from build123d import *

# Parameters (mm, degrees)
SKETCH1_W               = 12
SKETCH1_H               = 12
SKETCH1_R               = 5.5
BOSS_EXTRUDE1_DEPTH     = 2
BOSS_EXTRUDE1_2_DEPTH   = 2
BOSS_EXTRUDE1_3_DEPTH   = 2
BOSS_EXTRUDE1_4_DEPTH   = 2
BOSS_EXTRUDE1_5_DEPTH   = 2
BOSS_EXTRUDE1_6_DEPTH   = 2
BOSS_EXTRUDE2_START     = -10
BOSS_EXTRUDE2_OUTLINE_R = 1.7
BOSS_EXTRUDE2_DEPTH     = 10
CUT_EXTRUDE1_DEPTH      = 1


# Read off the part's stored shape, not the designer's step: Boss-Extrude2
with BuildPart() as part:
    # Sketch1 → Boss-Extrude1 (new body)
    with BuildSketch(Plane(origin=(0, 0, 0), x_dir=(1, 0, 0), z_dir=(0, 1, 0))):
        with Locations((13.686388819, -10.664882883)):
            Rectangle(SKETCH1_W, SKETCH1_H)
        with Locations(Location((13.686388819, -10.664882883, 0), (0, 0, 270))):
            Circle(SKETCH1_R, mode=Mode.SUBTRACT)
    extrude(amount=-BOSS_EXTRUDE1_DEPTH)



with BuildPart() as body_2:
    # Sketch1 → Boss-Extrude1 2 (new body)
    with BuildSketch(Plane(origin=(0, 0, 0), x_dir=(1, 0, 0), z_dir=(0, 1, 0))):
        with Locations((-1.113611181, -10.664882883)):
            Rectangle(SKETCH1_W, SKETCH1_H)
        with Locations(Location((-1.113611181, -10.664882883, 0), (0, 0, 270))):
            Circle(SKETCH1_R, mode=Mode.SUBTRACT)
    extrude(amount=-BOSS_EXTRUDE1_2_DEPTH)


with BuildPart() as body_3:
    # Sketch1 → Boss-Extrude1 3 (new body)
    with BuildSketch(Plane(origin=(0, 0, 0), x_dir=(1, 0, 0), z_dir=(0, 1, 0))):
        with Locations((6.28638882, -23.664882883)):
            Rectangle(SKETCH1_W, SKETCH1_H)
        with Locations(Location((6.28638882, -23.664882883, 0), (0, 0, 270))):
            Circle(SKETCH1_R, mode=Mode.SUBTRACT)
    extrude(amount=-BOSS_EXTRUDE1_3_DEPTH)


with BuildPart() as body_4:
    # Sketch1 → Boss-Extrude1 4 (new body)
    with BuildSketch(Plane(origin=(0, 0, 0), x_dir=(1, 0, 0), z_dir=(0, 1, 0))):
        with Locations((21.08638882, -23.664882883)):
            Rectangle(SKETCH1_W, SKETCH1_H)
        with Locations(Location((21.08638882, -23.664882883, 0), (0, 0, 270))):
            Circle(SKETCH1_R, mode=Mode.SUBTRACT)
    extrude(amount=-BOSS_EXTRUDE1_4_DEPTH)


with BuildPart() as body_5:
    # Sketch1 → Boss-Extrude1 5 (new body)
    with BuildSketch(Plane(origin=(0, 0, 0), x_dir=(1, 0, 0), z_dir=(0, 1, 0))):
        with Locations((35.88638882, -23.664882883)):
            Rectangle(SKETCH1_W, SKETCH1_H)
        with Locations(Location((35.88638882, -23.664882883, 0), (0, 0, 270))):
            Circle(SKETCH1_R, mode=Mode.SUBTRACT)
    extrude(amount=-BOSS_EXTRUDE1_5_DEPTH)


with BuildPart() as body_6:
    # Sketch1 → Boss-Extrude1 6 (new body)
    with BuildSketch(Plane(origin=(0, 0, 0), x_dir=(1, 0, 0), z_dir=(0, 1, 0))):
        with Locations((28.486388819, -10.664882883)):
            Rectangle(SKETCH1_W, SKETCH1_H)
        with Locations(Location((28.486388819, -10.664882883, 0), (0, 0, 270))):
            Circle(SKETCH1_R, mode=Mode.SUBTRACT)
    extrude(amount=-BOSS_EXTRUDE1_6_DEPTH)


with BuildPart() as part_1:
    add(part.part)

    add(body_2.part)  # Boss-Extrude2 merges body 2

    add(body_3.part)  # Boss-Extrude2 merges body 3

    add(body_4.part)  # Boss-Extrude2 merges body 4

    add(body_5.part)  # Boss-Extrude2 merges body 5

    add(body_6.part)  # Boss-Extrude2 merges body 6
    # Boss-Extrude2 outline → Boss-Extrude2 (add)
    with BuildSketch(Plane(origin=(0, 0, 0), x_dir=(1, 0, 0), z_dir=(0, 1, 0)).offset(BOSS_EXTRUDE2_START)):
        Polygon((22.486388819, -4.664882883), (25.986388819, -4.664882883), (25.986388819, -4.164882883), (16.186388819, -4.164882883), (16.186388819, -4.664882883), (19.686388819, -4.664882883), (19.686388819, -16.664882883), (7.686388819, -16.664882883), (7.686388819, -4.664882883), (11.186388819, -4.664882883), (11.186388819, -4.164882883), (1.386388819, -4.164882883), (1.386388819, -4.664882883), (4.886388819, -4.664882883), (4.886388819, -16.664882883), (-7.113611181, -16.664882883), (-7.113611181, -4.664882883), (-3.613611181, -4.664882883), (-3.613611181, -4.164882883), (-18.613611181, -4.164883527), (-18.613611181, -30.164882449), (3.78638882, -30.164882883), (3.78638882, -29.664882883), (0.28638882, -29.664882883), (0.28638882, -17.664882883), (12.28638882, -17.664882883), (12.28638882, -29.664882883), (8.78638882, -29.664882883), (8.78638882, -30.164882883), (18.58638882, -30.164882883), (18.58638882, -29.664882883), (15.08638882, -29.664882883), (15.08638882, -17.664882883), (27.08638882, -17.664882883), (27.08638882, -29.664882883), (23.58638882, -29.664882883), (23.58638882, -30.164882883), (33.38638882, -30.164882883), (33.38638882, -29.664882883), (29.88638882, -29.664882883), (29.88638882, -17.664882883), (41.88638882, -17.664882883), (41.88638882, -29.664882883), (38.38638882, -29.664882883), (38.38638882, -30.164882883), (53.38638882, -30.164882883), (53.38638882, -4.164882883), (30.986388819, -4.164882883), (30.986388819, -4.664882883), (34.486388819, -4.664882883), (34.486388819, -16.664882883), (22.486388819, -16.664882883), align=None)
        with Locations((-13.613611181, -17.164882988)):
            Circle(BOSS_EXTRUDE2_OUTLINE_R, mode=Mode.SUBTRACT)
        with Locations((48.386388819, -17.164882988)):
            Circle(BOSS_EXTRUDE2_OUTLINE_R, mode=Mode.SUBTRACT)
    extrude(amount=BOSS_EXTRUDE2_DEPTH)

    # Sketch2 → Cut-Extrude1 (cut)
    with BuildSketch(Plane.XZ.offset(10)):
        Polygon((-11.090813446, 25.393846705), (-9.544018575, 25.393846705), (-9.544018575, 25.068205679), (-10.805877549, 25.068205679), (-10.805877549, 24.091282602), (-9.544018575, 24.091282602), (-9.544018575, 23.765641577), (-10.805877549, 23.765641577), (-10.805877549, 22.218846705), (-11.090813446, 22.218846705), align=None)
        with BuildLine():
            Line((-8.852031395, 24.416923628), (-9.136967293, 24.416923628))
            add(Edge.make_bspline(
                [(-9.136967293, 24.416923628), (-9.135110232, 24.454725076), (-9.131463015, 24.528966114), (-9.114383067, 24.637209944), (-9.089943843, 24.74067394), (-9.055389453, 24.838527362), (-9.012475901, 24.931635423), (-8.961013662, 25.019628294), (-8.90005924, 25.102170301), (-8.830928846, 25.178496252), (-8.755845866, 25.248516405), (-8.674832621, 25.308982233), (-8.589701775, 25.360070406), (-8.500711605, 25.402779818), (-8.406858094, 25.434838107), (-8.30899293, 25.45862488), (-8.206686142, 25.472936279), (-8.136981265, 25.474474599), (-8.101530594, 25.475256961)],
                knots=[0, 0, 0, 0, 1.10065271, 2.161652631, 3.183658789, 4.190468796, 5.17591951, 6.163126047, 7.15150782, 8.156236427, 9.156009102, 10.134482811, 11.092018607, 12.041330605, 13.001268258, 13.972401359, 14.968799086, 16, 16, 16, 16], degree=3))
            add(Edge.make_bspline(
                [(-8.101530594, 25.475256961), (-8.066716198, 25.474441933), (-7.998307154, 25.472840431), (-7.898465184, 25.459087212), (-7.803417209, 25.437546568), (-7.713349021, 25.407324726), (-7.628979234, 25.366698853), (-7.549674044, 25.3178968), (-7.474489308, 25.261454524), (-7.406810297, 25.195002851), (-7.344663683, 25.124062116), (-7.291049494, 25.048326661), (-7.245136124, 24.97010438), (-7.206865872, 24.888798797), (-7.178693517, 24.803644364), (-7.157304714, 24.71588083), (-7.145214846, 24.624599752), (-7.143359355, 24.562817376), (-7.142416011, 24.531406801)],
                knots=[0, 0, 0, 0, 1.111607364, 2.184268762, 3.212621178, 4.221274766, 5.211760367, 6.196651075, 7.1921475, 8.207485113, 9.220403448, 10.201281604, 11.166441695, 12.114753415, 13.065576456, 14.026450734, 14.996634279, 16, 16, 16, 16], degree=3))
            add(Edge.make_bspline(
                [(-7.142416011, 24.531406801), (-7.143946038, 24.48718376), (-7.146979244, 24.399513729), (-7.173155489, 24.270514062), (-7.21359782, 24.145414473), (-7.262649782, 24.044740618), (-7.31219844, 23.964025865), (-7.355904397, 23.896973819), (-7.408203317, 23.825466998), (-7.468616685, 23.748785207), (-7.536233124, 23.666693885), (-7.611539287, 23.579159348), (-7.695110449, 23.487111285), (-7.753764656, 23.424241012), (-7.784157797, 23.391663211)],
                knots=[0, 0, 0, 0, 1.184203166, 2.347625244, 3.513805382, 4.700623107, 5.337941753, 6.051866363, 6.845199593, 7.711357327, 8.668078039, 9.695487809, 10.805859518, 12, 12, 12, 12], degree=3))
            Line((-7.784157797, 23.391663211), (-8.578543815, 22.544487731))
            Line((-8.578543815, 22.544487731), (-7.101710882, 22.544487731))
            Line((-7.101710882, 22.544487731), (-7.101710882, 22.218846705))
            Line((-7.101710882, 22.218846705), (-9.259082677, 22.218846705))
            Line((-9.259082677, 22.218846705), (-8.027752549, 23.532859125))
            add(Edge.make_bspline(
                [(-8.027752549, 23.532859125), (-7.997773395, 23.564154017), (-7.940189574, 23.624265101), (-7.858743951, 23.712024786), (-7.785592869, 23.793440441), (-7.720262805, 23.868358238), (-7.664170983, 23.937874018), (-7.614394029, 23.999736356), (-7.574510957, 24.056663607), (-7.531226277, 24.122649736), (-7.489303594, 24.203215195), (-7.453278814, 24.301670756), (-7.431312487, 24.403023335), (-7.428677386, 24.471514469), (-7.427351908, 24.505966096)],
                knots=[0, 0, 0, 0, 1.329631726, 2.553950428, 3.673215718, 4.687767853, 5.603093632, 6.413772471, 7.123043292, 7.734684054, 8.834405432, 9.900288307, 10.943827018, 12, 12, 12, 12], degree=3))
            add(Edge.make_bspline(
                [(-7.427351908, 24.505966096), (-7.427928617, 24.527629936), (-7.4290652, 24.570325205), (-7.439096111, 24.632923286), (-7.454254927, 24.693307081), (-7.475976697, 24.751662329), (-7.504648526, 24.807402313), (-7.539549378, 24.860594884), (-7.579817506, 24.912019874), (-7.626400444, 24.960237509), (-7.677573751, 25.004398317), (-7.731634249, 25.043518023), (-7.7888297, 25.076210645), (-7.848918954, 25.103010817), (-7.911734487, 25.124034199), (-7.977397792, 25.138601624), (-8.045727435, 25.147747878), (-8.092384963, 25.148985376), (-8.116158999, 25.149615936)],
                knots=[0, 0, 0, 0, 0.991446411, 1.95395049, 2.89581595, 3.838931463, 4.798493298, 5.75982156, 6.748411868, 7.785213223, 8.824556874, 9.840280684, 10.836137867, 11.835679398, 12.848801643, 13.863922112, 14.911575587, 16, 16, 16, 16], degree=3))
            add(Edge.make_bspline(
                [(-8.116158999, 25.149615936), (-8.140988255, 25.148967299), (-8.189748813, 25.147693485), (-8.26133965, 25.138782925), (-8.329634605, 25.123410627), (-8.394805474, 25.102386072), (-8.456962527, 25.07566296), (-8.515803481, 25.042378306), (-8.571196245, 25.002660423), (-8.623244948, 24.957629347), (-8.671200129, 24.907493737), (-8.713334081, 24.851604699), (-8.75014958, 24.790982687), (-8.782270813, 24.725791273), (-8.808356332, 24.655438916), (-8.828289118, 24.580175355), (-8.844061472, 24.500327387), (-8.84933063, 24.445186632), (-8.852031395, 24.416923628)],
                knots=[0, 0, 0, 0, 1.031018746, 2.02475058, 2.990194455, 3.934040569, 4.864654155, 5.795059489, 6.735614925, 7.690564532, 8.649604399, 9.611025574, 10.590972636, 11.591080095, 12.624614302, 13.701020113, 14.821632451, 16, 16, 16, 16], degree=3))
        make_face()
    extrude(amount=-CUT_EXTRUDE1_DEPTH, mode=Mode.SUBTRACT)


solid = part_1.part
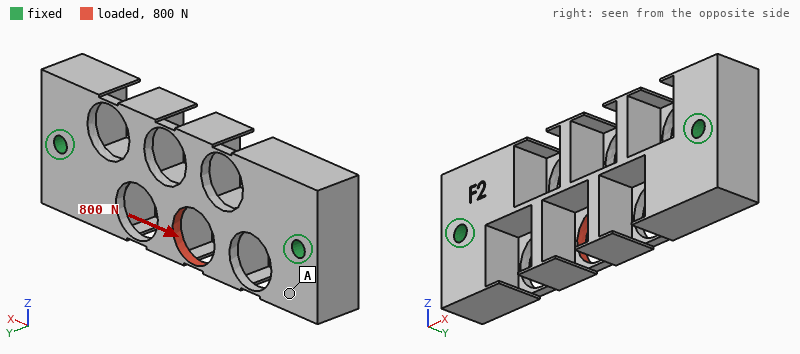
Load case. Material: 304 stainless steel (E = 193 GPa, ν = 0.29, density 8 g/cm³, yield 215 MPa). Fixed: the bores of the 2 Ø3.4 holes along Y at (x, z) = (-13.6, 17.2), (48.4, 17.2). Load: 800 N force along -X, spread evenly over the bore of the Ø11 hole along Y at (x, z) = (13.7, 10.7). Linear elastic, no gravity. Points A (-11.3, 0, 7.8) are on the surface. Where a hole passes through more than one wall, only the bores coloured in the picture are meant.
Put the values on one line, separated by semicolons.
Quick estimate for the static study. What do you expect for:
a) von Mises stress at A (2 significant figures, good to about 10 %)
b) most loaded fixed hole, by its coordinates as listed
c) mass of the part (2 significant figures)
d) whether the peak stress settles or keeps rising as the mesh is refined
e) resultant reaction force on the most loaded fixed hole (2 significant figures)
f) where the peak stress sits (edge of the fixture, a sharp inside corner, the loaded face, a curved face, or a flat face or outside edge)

8.6 MPa; (-13.6, 17.2); 83 g; keeps rising; 470 N; a sharp inside corner
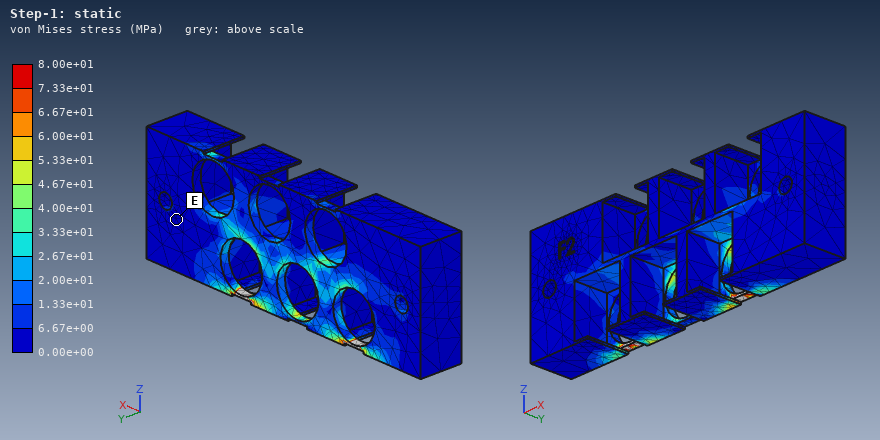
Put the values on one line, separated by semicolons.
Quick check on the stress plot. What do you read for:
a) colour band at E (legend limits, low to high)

0.00e+00 to 6.67e+00 MPa
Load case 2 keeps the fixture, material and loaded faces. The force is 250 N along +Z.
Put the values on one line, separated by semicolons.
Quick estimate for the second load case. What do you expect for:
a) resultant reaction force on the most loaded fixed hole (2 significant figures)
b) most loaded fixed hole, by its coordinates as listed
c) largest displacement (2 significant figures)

150 N; (-13.6, 17.2); 7.8 µm
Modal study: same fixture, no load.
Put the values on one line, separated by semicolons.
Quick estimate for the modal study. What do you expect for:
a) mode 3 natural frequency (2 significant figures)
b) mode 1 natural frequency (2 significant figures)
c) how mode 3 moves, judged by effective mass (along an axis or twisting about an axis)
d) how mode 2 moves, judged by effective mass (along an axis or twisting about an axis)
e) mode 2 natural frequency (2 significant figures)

8300 Hz; 5900 Hz; along Z; along Y; 7600 Hz
